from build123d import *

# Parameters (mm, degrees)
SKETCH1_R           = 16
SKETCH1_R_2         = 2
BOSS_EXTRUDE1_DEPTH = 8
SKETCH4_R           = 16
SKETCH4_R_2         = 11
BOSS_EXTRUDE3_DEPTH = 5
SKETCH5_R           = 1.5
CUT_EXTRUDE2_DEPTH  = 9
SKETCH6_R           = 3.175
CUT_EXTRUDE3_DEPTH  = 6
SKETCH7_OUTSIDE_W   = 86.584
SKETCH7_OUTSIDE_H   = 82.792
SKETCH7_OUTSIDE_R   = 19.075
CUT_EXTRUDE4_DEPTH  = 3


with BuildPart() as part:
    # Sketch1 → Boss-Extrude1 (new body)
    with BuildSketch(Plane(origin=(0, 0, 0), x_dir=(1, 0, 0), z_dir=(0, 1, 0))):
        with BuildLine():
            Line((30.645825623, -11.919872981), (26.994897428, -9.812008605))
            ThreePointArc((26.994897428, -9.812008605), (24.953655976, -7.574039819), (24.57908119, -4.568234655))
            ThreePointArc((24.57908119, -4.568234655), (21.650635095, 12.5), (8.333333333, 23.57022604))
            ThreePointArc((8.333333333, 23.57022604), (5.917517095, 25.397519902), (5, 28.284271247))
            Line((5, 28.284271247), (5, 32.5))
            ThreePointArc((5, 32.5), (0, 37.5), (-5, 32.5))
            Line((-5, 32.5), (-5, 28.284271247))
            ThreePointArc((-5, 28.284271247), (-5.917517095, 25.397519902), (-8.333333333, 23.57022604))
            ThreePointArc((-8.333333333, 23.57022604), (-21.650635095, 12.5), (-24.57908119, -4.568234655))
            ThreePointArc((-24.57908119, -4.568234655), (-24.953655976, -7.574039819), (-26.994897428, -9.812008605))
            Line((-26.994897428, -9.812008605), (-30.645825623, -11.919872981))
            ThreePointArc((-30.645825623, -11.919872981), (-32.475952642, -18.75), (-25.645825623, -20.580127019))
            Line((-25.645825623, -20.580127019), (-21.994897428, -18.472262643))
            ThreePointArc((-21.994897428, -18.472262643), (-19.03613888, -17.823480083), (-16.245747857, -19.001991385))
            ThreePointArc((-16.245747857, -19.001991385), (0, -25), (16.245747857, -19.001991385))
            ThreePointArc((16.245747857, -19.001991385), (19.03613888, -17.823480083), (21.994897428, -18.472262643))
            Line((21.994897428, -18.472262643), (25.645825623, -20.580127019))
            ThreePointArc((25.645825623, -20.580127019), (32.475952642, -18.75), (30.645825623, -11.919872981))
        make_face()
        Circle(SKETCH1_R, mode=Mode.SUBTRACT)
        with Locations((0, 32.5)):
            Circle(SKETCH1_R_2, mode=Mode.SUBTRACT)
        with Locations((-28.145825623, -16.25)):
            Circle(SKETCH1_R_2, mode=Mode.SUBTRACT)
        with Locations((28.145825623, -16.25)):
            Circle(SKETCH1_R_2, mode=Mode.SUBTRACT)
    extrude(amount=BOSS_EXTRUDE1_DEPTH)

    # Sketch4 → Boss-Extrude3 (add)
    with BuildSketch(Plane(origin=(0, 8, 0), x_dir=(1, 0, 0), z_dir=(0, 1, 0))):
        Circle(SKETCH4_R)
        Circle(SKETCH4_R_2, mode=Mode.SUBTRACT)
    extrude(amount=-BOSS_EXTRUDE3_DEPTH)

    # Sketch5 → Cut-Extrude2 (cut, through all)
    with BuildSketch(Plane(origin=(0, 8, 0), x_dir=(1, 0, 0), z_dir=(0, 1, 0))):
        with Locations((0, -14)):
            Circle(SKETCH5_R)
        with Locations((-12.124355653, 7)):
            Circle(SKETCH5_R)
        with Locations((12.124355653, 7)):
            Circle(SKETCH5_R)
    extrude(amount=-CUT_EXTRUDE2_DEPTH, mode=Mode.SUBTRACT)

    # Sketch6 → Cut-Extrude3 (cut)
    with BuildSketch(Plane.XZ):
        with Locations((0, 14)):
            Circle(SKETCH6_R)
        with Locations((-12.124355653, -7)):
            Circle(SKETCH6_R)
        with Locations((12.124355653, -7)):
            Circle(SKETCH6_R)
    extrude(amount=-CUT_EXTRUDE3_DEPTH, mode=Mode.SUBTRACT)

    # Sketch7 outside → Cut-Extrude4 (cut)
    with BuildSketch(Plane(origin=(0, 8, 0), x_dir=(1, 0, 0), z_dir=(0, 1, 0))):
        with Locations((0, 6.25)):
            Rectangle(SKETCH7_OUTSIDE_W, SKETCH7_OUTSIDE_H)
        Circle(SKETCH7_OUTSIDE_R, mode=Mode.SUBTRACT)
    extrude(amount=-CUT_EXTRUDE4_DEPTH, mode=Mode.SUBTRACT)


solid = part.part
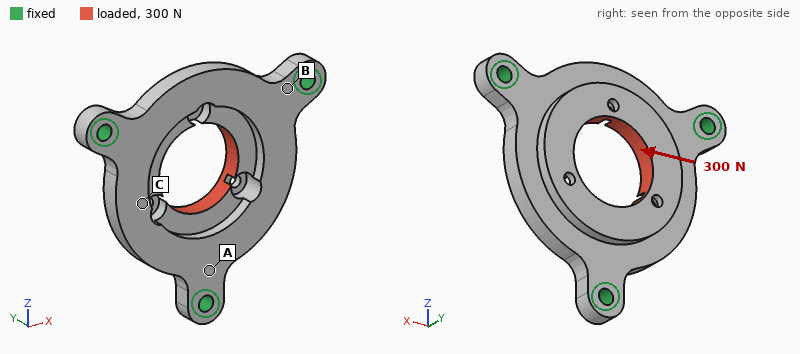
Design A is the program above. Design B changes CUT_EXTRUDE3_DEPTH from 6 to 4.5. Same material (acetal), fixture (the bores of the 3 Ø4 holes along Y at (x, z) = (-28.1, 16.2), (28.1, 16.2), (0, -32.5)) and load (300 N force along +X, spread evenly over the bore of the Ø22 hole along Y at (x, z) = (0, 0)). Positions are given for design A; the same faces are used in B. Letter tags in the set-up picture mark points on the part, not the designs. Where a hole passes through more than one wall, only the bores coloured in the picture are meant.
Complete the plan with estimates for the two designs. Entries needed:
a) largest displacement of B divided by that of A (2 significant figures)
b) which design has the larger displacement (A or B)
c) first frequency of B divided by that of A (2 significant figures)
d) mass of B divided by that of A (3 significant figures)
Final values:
0.81
A
1.0
1.01
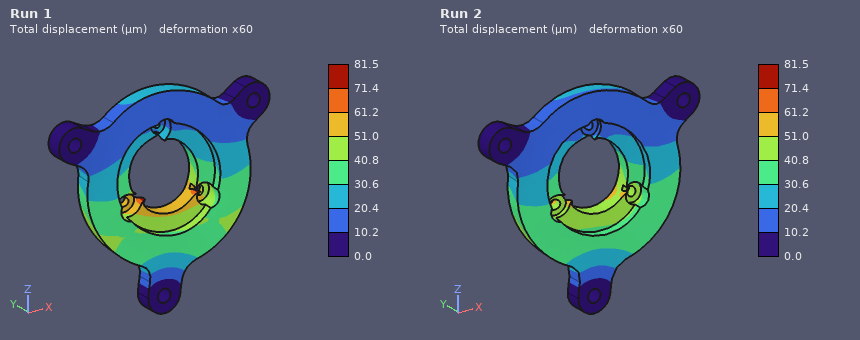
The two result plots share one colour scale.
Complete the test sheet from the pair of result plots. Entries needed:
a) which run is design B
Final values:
Run 2
